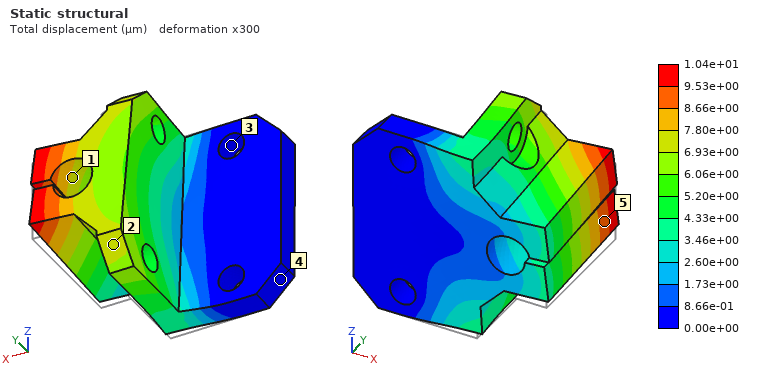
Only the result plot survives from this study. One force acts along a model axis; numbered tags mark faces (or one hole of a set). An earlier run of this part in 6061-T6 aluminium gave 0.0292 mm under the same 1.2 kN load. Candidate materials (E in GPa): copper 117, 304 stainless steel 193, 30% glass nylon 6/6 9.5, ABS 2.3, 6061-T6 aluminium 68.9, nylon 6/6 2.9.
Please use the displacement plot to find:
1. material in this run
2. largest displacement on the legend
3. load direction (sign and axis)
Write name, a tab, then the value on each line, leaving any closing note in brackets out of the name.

material in this run	304 stainless steel
largest displacement on the legend	1.04e+01 µm
load direction	+Z
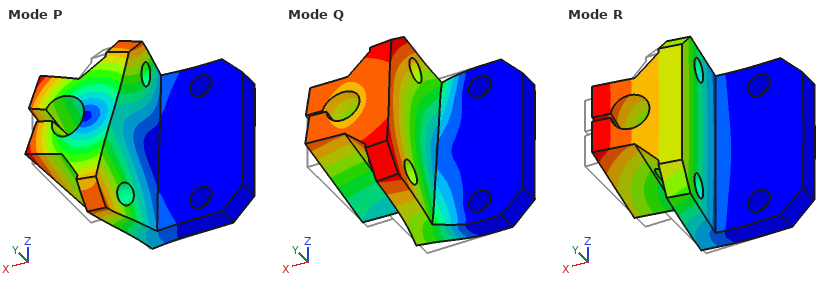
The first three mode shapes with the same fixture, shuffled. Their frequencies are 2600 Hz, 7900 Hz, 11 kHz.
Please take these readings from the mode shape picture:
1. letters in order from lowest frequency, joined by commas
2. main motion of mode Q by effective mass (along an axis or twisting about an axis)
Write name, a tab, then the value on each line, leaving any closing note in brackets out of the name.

letters in order from lowest frequency, joined by commas	R, Q, P
main motion of mode Q by effective mass	along Z
